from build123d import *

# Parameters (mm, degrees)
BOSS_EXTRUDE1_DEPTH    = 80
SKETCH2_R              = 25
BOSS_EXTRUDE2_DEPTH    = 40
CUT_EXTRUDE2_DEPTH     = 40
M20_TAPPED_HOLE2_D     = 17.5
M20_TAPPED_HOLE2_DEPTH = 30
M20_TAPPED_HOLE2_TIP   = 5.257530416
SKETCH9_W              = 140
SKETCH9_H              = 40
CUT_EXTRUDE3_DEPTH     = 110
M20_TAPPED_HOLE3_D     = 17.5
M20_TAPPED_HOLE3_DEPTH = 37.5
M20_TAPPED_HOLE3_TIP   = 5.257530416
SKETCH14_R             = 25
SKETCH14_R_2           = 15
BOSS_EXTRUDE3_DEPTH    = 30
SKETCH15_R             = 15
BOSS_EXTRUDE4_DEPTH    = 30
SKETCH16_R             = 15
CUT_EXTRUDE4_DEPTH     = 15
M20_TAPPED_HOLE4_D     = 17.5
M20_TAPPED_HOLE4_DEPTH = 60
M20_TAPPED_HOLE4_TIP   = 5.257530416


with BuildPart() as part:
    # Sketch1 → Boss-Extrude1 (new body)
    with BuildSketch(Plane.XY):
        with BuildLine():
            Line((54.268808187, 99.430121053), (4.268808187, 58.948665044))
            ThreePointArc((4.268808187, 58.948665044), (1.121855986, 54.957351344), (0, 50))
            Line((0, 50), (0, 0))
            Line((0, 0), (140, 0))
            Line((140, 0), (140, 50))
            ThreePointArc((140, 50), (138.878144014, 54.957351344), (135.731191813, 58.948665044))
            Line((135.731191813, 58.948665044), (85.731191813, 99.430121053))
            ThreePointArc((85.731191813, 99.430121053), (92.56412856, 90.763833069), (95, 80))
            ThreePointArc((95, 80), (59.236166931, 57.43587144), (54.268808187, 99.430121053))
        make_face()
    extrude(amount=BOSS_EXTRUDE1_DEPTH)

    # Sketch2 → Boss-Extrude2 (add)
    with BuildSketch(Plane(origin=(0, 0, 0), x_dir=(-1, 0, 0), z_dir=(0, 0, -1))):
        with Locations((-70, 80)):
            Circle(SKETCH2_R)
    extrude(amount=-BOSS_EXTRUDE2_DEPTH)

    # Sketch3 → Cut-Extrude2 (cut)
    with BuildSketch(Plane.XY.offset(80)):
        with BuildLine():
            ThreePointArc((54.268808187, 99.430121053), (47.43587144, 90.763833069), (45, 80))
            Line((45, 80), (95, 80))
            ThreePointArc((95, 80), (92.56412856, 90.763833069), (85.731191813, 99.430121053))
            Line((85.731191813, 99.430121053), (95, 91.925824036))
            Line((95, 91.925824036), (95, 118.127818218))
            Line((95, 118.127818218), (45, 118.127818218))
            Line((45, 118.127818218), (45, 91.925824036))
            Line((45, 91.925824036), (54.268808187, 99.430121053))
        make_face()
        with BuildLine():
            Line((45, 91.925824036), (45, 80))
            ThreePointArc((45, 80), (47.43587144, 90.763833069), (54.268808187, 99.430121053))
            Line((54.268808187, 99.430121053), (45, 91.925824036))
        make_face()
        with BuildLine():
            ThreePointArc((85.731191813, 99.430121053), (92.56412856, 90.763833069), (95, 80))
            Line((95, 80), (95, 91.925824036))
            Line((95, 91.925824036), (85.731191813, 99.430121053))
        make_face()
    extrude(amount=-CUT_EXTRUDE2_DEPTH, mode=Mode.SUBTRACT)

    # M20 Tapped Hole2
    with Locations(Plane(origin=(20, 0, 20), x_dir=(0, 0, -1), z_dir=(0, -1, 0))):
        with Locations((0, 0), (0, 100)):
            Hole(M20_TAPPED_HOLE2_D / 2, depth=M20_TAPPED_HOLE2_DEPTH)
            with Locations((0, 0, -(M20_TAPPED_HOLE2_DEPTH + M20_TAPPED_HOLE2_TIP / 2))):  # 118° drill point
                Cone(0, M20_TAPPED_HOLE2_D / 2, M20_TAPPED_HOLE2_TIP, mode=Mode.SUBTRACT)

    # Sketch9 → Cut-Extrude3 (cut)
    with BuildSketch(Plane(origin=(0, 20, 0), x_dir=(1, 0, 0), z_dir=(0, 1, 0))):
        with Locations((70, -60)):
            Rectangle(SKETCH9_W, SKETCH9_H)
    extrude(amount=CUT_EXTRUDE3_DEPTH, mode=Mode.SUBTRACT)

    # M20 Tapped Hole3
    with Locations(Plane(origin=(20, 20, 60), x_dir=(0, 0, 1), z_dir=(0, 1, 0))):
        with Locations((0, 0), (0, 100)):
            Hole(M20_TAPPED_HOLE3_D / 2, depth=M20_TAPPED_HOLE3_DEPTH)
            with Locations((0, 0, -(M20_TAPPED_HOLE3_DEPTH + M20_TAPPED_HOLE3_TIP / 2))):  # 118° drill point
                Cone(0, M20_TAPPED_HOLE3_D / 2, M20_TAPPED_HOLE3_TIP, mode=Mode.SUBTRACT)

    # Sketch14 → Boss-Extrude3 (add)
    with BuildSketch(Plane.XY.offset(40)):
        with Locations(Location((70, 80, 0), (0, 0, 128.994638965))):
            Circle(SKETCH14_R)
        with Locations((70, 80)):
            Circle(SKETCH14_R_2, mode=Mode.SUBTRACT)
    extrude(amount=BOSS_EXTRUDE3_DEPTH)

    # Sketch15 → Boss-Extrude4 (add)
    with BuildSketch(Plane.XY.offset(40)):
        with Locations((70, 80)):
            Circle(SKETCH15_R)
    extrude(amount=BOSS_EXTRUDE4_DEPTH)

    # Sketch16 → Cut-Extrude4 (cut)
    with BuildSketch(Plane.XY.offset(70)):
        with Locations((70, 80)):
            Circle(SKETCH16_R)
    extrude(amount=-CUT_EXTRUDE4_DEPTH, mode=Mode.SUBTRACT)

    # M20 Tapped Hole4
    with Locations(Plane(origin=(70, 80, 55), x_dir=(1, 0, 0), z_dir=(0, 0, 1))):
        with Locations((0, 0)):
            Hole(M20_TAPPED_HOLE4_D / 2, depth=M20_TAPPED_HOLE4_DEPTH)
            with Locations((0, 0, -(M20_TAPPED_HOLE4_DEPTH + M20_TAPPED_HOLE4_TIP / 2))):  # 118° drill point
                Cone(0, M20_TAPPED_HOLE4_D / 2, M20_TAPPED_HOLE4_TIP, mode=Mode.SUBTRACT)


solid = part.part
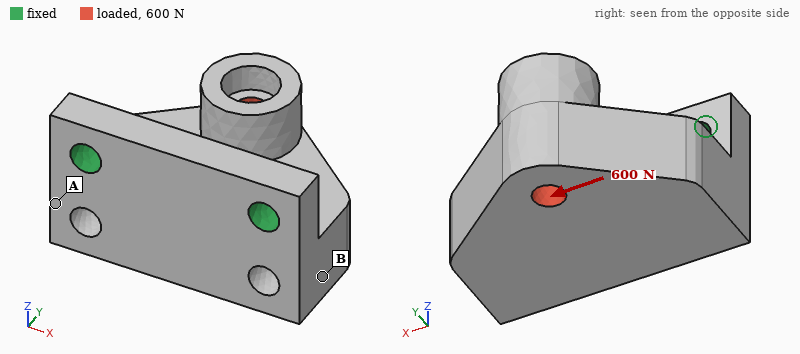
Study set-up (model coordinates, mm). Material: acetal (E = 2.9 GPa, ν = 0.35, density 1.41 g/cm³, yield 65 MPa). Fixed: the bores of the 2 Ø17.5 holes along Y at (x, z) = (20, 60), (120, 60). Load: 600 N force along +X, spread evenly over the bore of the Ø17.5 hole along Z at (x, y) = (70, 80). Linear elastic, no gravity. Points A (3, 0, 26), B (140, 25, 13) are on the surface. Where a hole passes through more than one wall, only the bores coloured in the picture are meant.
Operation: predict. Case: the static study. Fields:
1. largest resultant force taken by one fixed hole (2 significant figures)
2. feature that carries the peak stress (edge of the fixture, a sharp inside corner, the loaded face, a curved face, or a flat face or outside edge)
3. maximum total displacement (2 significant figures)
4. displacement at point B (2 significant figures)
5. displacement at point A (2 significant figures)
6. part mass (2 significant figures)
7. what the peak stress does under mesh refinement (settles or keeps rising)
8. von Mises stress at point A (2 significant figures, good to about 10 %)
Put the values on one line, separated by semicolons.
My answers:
520 N; edge of the fixture; 76 µm; 39 µm; 29 µm; 830 g; keeps rising; 0.63 MPa
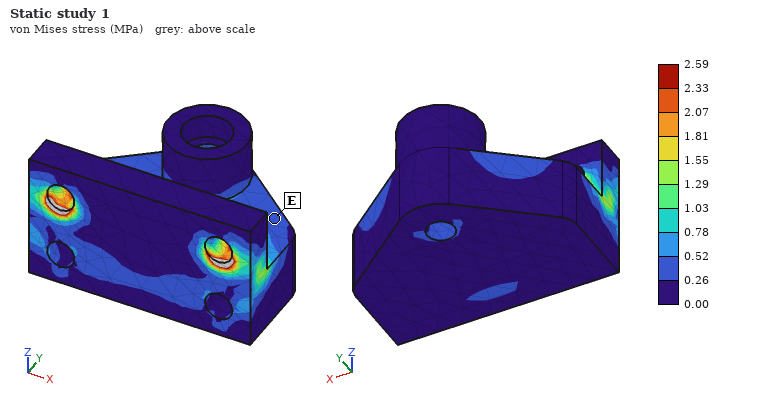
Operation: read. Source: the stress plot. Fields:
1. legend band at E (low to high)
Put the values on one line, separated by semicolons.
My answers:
0.26 to 0.52 MPa
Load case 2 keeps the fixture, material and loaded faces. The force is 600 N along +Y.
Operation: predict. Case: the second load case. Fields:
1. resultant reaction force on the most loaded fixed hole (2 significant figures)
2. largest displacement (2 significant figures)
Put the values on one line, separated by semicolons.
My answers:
300 N; 0.13 mm
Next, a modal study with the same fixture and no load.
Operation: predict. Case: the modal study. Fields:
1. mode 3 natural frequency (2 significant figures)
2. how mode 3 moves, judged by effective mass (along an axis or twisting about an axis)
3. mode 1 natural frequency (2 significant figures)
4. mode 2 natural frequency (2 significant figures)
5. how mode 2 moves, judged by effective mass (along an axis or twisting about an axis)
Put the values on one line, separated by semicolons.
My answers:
1200 Hz; along Y; 330 Hz; 870 Hz; along X
